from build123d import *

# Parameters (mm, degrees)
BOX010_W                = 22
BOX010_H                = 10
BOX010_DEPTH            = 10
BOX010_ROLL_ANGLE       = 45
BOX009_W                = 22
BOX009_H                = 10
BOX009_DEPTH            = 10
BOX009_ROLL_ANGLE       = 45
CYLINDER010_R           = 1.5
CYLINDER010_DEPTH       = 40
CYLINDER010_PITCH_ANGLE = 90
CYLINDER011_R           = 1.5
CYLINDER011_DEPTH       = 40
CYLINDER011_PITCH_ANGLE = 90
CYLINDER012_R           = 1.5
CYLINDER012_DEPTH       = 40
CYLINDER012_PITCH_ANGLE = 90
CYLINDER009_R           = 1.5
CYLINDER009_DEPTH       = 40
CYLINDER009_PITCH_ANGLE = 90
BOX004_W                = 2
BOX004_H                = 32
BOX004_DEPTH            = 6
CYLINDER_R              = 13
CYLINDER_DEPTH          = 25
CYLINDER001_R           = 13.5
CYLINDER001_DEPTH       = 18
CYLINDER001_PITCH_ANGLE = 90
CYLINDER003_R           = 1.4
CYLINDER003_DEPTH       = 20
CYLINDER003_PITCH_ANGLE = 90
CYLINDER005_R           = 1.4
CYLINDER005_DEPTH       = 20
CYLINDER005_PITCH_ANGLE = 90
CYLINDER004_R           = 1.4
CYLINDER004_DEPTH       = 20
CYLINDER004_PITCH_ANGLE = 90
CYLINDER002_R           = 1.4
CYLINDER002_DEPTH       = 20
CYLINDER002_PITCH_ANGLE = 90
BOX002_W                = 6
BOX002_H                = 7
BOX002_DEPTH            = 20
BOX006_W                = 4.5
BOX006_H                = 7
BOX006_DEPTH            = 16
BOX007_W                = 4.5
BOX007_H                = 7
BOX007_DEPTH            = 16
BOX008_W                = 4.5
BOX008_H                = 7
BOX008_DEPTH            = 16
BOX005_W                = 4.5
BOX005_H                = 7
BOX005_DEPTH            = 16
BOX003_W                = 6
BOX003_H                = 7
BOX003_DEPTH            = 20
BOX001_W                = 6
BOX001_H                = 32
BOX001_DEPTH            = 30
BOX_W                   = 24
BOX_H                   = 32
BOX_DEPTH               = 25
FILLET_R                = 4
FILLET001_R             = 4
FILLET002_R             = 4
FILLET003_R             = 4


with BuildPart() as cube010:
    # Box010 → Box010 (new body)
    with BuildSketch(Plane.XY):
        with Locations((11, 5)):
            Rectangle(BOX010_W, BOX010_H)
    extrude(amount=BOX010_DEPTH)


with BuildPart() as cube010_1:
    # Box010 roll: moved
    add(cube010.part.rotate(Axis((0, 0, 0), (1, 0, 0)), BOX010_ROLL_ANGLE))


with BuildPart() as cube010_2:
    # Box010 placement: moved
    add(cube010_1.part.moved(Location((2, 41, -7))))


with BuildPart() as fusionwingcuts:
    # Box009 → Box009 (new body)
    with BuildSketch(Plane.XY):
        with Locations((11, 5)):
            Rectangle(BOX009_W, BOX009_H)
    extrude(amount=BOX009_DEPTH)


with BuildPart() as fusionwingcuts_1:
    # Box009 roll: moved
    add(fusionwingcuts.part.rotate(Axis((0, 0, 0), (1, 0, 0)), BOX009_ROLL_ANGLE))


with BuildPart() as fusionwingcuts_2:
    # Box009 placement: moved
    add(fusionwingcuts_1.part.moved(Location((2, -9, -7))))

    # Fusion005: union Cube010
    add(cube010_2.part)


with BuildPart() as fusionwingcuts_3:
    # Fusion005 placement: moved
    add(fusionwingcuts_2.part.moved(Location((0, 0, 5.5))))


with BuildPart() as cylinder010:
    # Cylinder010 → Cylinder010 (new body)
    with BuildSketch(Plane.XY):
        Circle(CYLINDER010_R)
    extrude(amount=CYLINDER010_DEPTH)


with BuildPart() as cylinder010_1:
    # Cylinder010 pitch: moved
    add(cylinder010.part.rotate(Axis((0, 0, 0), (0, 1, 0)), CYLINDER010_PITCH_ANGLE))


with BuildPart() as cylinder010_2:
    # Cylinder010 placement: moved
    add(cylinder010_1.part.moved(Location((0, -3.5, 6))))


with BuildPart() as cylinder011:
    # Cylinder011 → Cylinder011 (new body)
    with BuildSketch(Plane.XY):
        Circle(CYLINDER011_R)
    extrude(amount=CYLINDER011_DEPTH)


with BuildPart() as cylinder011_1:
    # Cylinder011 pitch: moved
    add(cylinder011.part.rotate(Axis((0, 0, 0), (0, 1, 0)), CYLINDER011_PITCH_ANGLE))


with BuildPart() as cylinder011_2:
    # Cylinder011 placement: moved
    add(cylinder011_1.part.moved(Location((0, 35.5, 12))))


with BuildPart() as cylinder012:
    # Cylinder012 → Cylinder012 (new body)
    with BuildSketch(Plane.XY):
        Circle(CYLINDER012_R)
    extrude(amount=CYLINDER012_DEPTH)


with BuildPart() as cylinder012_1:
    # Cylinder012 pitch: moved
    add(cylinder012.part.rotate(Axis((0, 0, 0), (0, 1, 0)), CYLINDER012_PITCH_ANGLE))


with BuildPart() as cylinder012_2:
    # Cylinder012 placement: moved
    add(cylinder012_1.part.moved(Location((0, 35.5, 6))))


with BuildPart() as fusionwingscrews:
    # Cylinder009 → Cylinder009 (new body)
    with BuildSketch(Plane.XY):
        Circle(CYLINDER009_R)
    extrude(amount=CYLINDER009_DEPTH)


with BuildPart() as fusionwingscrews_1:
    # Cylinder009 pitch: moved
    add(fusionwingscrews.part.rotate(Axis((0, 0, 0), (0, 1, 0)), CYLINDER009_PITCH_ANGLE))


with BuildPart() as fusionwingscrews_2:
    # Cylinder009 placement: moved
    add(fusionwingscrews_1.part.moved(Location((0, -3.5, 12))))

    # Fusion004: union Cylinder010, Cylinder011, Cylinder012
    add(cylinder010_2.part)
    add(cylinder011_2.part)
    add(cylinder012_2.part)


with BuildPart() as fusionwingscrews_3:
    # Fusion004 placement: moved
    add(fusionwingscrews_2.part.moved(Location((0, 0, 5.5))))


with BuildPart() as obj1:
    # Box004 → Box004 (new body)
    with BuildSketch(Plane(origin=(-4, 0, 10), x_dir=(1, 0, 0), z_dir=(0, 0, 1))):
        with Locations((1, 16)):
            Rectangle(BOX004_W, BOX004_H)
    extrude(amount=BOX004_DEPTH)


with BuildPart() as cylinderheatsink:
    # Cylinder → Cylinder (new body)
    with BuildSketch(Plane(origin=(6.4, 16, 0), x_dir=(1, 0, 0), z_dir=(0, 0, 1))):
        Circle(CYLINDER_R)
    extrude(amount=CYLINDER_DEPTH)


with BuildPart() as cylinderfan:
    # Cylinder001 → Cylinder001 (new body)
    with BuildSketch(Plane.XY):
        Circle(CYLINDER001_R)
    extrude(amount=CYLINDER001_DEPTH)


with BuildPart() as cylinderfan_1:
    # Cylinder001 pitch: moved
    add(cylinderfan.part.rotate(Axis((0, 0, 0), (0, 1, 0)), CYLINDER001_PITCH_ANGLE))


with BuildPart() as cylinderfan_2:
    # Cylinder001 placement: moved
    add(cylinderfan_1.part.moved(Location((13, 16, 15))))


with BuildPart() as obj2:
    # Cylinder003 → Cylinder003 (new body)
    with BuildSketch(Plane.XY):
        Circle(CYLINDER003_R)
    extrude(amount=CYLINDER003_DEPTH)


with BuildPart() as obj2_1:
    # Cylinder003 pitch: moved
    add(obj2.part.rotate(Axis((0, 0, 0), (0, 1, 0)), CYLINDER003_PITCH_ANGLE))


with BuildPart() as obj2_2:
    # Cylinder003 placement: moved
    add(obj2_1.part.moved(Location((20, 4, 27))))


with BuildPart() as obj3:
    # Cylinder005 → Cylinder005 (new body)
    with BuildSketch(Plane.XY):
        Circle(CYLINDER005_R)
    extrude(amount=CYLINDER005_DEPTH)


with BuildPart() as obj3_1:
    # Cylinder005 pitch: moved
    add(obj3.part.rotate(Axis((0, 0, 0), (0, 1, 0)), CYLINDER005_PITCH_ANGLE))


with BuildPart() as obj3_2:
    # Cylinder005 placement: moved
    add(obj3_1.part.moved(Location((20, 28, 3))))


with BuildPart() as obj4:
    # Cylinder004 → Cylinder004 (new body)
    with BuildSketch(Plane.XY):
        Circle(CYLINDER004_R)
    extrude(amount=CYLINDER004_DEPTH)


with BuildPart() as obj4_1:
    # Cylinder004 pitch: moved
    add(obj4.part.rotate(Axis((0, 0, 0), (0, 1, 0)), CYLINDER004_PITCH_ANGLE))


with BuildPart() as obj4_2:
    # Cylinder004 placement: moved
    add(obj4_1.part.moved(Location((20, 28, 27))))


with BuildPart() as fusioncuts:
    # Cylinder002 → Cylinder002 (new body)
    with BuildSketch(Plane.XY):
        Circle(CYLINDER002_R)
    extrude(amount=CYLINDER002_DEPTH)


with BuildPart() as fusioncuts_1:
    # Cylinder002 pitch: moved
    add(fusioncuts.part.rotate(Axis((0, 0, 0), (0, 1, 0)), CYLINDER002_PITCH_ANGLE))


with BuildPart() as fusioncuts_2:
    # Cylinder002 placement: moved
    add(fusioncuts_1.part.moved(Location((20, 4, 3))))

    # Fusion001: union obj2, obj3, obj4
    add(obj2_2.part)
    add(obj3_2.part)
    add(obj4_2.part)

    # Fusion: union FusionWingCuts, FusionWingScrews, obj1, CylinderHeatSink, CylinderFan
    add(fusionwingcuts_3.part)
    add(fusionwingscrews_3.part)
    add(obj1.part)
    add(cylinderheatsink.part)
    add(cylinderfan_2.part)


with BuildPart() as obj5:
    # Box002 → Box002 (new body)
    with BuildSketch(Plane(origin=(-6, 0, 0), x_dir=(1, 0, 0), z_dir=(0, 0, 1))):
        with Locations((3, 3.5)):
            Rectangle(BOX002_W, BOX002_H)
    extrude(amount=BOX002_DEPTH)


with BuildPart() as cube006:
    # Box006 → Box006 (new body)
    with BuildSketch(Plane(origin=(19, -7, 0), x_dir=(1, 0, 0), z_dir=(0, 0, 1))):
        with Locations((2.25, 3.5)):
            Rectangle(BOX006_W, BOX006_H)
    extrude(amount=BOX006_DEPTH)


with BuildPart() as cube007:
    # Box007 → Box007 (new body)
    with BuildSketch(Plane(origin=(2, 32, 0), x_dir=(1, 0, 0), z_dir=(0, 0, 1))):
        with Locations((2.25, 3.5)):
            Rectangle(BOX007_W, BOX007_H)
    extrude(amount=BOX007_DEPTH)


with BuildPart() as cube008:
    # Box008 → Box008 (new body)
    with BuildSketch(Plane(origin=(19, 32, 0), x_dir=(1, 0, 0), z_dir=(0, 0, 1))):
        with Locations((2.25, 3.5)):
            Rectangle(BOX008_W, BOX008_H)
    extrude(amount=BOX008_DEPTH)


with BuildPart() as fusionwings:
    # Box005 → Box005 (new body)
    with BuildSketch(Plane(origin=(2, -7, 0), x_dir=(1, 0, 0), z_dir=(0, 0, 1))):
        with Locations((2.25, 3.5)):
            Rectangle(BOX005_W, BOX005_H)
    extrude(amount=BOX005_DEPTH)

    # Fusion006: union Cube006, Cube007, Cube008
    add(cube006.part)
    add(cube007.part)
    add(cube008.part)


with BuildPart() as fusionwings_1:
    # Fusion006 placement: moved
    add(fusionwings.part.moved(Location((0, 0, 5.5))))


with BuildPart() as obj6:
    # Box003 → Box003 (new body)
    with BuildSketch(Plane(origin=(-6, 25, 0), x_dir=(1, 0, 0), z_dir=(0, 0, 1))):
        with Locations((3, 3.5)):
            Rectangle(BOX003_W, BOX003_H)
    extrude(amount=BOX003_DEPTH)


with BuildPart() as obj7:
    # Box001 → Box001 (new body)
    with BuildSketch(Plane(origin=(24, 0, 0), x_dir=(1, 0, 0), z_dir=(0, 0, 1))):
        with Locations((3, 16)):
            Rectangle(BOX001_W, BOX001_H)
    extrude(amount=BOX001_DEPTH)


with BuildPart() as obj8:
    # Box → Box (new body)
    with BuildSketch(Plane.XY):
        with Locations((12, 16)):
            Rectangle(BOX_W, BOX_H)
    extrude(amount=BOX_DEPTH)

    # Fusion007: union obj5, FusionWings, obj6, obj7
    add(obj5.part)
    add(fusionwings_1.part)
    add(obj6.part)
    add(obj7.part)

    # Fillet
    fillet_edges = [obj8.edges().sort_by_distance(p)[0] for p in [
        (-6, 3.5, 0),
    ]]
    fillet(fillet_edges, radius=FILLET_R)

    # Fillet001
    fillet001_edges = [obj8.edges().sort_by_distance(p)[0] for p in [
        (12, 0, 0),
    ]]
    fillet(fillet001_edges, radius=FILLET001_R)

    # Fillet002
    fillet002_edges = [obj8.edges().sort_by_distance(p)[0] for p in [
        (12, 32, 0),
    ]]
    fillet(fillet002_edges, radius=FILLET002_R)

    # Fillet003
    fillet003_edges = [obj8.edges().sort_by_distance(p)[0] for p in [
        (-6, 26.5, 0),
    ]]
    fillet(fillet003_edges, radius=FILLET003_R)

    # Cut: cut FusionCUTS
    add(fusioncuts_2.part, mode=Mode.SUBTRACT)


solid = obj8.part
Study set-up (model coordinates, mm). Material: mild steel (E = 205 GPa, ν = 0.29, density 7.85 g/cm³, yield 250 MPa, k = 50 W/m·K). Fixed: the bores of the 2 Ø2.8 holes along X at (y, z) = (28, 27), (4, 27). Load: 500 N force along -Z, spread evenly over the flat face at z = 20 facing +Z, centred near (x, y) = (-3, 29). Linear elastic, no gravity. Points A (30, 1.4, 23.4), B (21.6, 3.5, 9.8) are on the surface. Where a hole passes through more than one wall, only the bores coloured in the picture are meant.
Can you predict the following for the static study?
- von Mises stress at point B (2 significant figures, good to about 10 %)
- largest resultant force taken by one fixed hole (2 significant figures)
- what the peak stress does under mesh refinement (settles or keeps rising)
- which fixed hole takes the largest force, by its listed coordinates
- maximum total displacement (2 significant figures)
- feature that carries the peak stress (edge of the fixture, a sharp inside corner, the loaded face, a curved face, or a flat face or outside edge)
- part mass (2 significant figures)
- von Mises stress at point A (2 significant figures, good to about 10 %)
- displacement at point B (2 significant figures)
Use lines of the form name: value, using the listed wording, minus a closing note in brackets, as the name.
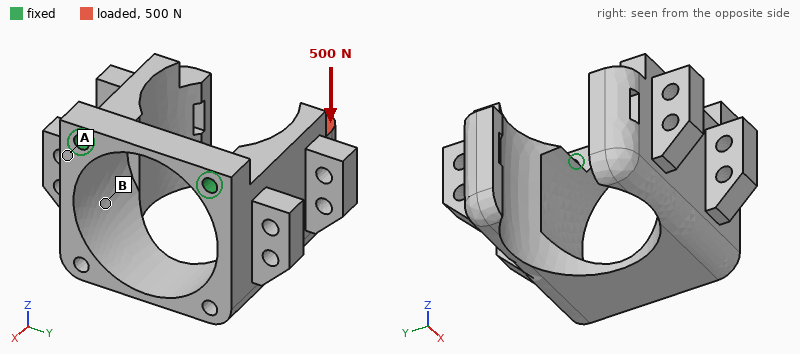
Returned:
von Mises stress at point B: 23 MPa
largest resultant force taken by one fixed hole: 490 N
what the peak stress does under mesh refinement: keeps rising
which fixed hole takes the largest force, by its listed coordinates: (28, 27)
maximum total displacement: 0.13 mm
feature that carries the peak stress: a sharp inside corner
part mass: 76 g
von Mises stress at point A: 100 MPa
displacement at point B: 0.021 mm
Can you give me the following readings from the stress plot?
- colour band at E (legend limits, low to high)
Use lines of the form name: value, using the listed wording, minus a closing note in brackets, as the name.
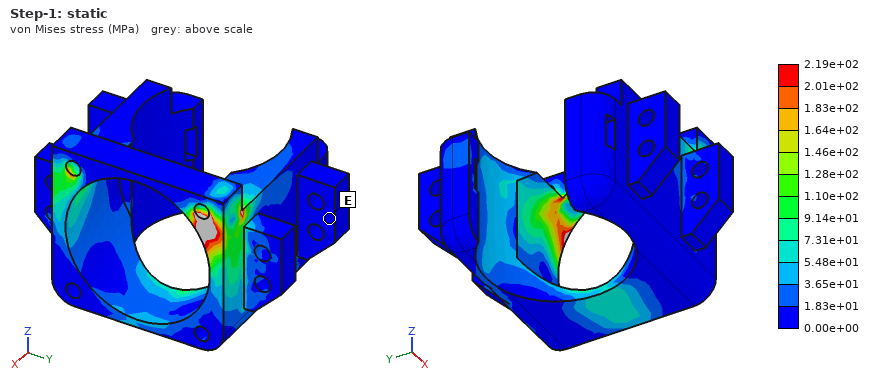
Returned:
colour band at E: 0.00e+00 to 1.83e+01 MPa
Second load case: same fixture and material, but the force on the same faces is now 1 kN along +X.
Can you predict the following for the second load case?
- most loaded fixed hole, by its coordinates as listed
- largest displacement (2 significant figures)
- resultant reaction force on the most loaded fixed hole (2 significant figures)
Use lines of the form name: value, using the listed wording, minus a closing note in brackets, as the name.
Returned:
most loaded fixed hole, by its coordinates as listed: (28, 27)
largest displacement: 38 µm
resultant reaction force on the most loaded fixed hole: 950 N
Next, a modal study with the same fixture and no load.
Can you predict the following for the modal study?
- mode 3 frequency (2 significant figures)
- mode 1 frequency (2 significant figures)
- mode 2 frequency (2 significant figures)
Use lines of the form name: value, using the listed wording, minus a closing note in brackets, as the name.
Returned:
mode 3 frequency: 3200 Hz
mode 1 frequency: 2200 Hz
mode 2 frequency: 2300 Hz
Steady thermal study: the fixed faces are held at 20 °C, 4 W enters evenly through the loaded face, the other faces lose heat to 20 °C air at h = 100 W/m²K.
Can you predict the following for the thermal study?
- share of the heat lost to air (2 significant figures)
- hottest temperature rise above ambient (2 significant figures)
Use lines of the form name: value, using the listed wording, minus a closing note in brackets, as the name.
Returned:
share of the heat lost to air: 74 %
hottest temperature rise above ambient: 30 K
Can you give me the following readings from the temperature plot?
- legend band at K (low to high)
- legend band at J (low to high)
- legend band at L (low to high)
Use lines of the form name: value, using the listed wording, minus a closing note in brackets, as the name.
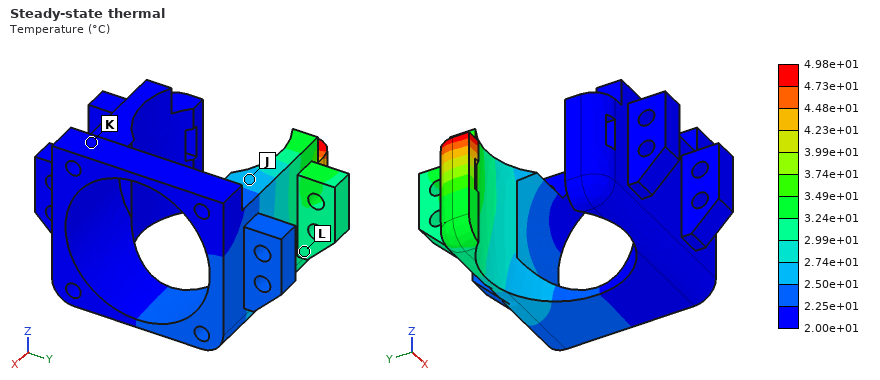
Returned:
legend band at K: 2.00e+01 to 2.25e+01 °C
legend band at J: 2.50e+01 to 2.74e+01 °C
legend band at L: 2.99e+01 to 3.24e+01 °C
